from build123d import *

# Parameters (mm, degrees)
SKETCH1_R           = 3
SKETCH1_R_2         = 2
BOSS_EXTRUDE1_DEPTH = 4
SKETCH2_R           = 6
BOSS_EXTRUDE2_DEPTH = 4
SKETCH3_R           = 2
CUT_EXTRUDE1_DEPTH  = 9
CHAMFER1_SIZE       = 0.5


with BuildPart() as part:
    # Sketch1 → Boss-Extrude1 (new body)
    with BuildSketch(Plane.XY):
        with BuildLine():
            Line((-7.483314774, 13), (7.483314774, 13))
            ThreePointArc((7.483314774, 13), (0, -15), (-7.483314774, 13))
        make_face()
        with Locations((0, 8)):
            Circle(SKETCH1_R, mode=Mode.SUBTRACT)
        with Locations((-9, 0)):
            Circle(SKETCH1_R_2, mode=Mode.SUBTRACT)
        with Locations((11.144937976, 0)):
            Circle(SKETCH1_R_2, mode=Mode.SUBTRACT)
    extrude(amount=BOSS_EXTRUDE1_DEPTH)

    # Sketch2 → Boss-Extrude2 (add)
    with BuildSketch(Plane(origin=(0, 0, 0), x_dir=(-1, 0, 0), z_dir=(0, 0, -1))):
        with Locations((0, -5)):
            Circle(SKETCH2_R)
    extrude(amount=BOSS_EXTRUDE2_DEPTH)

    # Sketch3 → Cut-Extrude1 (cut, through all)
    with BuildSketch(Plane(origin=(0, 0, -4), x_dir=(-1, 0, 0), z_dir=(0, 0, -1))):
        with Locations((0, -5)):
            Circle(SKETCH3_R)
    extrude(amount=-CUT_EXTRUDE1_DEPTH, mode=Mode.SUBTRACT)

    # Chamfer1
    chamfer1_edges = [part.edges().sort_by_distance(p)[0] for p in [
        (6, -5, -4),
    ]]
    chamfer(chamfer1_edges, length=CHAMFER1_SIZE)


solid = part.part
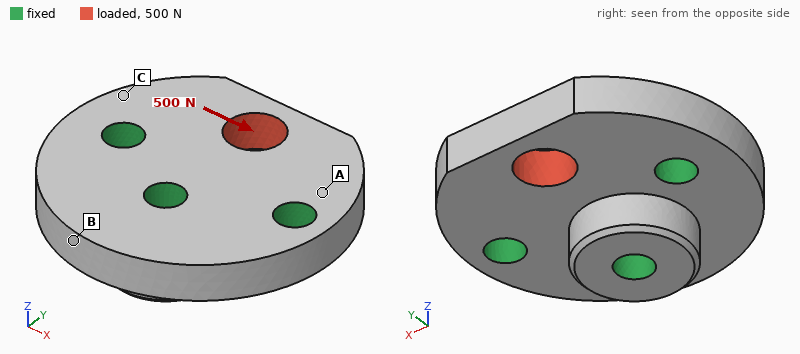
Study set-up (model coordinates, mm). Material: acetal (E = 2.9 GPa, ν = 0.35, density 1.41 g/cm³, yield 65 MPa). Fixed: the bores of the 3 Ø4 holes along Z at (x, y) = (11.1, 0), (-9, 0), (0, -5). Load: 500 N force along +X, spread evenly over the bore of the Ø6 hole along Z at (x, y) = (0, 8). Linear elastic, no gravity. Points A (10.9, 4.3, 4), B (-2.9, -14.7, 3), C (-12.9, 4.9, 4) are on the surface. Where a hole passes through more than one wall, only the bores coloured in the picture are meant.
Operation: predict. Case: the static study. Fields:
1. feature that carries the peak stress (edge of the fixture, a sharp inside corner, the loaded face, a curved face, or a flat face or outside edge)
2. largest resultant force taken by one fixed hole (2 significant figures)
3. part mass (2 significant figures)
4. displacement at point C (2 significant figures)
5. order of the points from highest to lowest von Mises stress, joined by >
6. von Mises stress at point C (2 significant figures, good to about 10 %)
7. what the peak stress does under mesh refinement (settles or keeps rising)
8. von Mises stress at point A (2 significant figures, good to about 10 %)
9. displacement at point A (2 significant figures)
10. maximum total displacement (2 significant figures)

edge of the fixture
290 N
4.1 g
26 µm
A > C > B
4.6 MPa
keeps rising
7.3 MPa
16 µm
73 µm
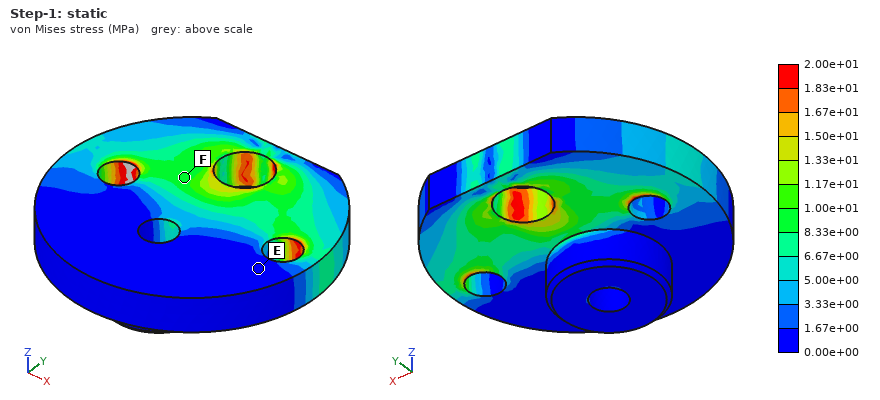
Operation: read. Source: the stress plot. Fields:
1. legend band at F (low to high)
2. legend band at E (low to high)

8.33e+00 to 1.00e+01 MPa
0.00e+00 to 1.67e+00 MPa
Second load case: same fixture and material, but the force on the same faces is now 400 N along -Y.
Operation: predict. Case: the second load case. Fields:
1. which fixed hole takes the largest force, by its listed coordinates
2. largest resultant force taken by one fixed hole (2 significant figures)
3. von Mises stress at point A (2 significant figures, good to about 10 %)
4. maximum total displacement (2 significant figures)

(0, -5)
180 N
2.5 MPa
51 µm
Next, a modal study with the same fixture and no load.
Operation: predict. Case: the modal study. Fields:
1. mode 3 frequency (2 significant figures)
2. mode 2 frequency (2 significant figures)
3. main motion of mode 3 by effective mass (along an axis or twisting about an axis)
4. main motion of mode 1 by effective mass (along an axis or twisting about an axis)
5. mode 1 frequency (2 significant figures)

15 kHz
10 kHz
along Z
along Z
6300 Hz
